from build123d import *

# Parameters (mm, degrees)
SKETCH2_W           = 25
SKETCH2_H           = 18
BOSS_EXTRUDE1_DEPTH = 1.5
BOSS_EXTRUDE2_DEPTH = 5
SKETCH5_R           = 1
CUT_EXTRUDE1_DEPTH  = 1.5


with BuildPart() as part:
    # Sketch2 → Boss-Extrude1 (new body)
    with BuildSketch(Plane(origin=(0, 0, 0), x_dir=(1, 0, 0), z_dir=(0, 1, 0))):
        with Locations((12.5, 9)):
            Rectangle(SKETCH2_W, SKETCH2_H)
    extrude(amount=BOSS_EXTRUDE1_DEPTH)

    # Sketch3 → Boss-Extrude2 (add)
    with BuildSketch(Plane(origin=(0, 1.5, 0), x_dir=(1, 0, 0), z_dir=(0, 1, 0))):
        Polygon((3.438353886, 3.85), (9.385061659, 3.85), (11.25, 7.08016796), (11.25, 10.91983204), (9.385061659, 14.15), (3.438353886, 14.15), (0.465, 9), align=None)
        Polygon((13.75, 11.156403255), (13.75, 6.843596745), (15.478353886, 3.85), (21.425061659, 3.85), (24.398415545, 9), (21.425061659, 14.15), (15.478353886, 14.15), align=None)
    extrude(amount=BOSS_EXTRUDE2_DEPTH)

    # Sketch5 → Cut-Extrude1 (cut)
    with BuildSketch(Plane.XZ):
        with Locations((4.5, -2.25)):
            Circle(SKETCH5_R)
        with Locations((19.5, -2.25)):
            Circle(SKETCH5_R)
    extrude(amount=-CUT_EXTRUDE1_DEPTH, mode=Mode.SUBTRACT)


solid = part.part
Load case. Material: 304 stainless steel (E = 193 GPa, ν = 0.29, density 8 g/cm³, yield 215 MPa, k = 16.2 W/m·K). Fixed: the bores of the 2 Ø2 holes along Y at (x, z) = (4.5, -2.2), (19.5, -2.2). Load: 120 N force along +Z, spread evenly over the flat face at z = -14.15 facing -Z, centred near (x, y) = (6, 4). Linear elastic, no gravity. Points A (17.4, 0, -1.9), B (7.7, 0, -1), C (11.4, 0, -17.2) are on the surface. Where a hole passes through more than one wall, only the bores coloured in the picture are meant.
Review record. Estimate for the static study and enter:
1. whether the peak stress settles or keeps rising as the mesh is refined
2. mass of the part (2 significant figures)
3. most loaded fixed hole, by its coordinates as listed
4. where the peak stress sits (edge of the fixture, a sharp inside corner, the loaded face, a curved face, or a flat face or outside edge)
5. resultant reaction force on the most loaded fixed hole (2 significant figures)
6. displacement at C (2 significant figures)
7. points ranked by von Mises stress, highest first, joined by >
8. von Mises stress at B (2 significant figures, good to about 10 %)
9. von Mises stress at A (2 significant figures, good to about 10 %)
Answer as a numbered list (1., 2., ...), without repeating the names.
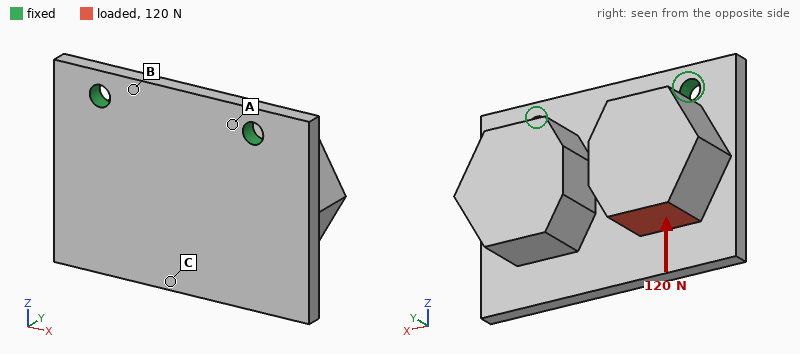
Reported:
1. keeps rising
2. 12 g
3. (4.5, -2.2)
4. edge of the fixture
5. 100 N
6. 13 µm
7. A > B > C
8. 17 MPa
9. 24 MPa
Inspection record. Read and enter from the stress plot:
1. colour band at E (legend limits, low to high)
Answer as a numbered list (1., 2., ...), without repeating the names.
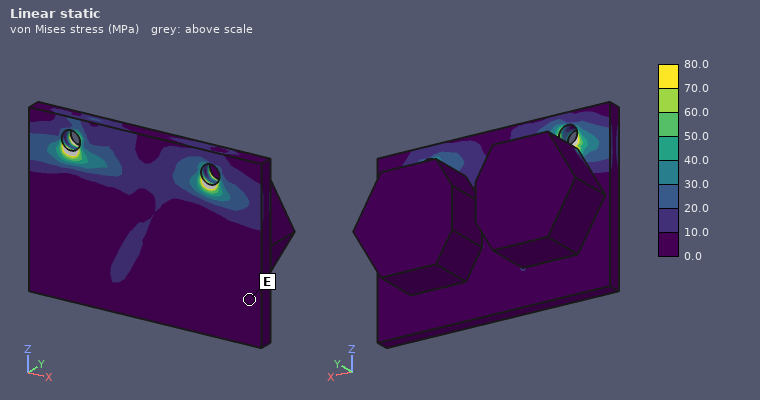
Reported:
1. 0.0 to 10.0 MPa
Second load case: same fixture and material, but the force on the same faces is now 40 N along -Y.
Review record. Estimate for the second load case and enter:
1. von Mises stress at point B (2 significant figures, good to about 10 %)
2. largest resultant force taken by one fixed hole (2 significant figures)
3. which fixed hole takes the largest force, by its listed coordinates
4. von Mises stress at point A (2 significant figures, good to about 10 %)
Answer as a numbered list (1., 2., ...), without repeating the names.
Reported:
1. 21 MPa
2. 30 N
3. (4.5, -2.2)
4. 29 MPa
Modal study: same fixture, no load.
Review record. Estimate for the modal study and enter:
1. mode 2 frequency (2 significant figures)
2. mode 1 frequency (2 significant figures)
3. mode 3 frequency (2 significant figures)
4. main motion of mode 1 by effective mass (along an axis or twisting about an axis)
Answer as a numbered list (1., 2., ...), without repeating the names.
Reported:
1. 11 kHz
2. 4000 Hz
3. 14 kHz
4. along Y
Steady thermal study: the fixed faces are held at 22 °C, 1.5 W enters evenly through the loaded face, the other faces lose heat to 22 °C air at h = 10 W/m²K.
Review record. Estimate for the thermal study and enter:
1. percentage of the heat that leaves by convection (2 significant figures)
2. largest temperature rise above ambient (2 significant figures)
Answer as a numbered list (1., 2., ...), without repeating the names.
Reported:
1. 10 %
2. 29 K
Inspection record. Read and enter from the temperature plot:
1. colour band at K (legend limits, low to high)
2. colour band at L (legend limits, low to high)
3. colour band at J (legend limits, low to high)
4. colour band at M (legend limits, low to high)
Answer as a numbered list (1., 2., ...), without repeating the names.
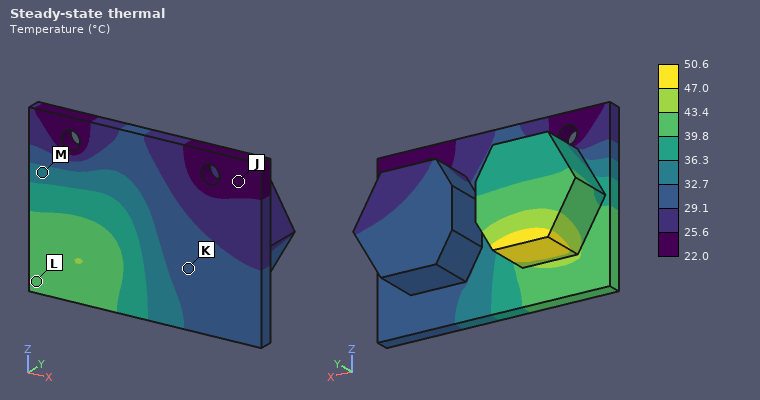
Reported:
1. 29.1 to 32.7 °C
2. 39.8 to 43.4 °C
3. 22.0 to 25.6 °C
4. 32.7 to 36.3 °C
